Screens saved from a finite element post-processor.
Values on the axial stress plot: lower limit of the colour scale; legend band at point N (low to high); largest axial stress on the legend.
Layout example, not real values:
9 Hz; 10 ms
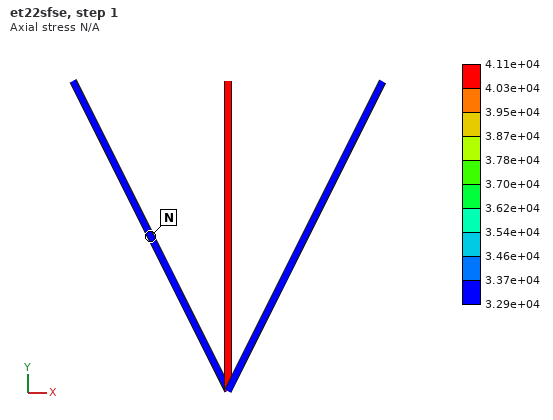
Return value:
3.29e+04; 3.29e+04 to 3.37e+04; 4.11e+04
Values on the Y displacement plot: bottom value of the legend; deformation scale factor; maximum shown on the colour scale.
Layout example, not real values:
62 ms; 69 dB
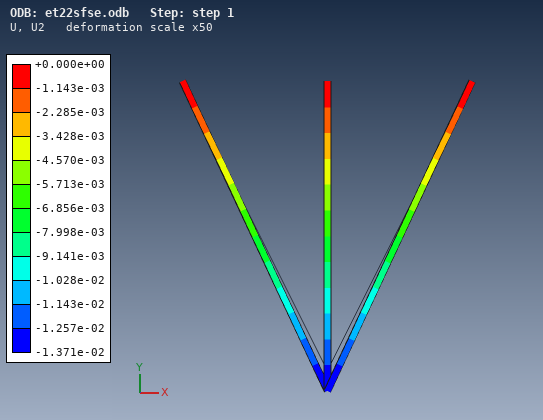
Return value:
-1.371e-02; 50; +0.000e+00
